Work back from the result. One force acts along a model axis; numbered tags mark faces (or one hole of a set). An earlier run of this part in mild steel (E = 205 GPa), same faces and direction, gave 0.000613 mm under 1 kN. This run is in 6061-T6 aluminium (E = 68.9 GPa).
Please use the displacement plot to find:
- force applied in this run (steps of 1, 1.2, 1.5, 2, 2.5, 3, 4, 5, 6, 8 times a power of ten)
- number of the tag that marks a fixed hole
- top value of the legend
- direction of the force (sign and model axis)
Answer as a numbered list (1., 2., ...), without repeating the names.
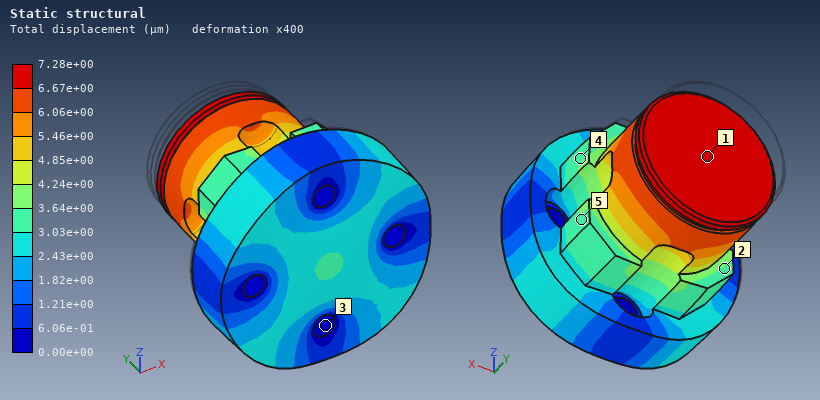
1. 4 kN
2. 3
3. 7.28e+00 µm
4. -Y
